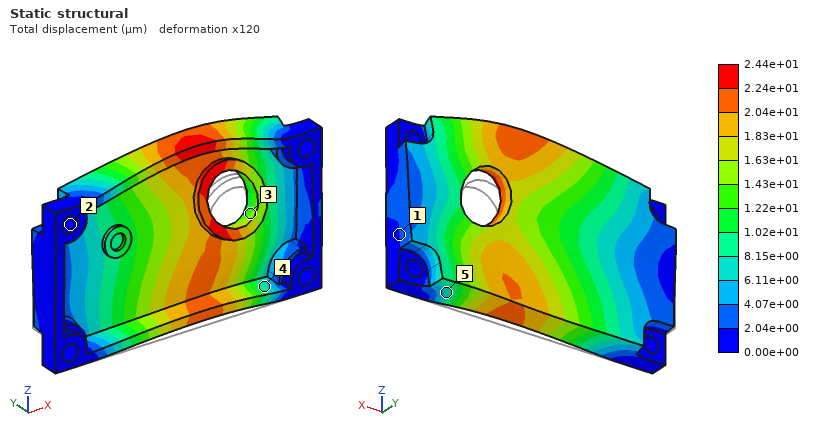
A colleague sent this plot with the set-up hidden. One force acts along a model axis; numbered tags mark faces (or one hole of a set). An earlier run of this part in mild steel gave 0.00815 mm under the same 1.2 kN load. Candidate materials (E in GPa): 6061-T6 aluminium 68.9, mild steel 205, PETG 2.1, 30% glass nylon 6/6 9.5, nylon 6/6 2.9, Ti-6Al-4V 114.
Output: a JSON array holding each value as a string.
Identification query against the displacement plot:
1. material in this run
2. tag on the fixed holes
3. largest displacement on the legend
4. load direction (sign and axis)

["6061-T6 aluminium", "2", "2.44e+01 µm", "+Z"]
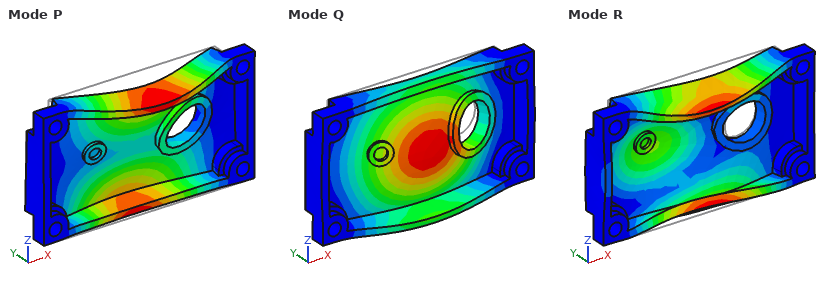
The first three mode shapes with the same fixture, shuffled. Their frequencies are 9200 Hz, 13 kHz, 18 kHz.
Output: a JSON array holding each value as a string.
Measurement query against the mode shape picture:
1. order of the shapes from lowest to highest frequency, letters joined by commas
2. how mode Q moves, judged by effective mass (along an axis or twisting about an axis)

["Q, P, R", "along Y"]
